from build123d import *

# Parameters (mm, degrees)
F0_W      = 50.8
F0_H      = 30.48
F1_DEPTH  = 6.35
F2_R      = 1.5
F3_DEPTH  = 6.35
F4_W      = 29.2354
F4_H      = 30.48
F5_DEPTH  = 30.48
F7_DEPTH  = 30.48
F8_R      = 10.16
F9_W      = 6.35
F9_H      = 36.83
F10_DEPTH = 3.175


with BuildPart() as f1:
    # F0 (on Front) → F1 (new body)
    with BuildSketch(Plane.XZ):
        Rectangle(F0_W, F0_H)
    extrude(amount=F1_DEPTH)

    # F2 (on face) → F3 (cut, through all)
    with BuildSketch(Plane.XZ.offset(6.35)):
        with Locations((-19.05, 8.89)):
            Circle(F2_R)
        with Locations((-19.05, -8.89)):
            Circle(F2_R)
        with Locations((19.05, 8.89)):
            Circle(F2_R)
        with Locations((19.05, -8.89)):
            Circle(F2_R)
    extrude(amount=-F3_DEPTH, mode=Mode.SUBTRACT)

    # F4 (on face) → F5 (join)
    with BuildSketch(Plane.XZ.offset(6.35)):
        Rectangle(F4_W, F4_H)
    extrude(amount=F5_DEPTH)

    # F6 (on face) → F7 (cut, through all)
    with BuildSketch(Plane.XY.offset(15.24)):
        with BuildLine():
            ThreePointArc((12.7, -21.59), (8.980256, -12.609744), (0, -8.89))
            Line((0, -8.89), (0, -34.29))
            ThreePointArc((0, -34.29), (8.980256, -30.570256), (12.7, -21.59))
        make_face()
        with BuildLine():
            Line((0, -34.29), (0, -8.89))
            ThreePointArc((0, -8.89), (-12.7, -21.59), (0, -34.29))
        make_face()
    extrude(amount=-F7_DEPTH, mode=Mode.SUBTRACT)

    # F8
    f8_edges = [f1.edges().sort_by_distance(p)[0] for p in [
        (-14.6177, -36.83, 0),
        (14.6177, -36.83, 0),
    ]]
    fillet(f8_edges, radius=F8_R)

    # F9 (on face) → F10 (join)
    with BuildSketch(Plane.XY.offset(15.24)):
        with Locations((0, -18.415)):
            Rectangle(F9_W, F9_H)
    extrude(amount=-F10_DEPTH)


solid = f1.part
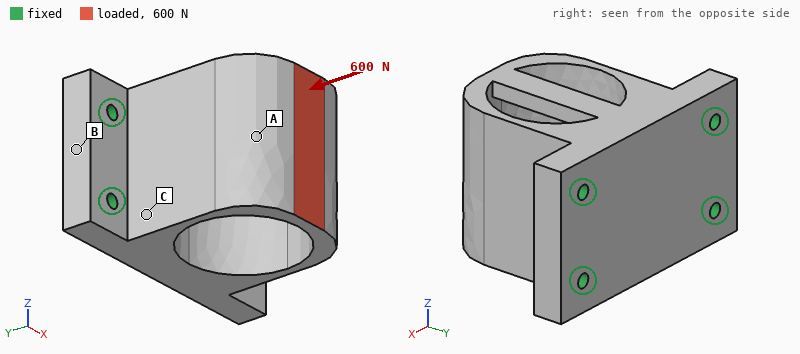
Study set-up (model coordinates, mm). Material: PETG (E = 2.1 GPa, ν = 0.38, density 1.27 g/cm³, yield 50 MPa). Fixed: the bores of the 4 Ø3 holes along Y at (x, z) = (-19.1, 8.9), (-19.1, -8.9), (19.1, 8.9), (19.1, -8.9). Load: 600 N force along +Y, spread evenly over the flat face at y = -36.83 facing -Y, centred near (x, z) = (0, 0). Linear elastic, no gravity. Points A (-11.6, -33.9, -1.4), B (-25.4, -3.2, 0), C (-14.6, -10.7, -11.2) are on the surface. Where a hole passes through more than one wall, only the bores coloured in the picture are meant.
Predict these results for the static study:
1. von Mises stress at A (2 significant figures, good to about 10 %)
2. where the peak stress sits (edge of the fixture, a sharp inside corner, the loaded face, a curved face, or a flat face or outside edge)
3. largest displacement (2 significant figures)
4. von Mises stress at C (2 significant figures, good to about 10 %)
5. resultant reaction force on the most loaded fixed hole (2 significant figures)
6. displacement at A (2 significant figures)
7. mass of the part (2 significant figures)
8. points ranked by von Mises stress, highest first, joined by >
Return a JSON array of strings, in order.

["6.1 MPa", "the loaded face", "0.58 mm", "11 MPa", "150 N", "0.13 mm", "26 g", "C > A > B"]
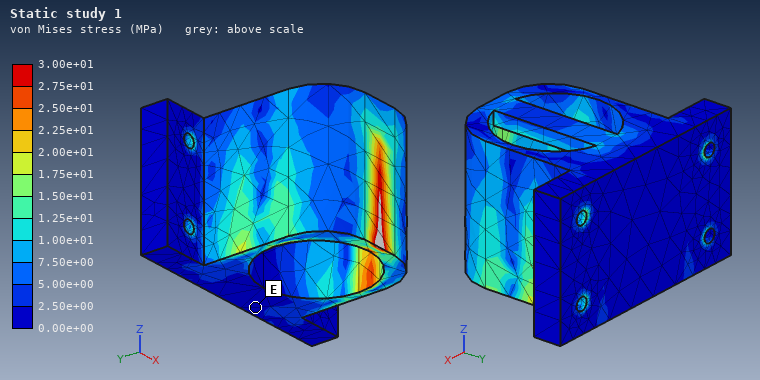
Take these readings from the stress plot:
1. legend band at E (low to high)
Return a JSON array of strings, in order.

["0.00e+00 to 2.50e+00 MPa"]
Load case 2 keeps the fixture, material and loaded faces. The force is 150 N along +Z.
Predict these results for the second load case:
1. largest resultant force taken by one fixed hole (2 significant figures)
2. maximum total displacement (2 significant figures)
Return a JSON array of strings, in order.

["130 N", "0.24 mm"]
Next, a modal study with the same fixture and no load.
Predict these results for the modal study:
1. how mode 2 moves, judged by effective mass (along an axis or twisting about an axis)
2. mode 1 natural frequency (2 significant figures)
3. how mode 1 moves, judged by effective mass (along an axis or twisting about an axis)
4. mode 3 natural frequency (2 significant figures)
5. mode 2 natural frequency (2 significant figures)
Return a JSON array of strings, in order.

["along Z", "1500 Hz", "along X", "3400 Hz", "2000 Hz"]
